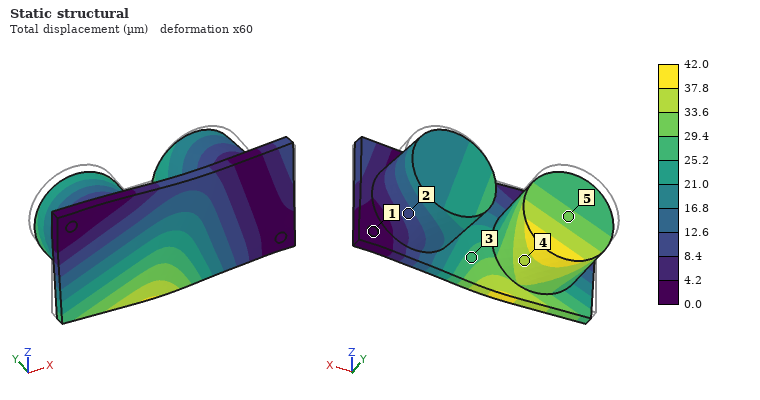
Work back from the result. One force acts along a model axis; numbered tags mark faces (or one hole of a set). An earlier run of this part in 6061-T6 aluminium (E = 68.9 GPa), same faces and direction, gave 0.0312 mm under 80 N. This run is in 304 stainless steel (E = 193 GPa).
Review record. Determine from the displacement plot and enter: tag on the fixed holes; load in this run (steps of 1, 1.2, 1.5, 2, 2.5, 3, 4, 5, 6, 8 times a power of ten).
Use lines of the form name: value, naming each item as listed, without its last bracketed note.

tag on the fixed holes: 1
load in this run: 300 N
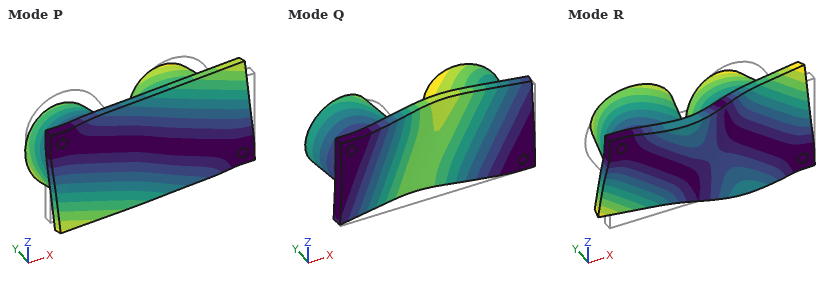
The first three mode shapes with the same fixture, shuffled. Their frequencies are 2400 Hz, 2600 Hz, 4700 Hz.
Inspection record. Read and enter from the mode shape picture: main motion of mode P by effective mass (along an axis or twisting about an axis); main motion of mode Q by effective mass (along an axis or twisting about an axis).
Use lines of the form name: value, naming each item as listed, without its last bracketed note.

main motion of mode P by effective mass: along Z
main motion of mode Q by effective mass: along Y
